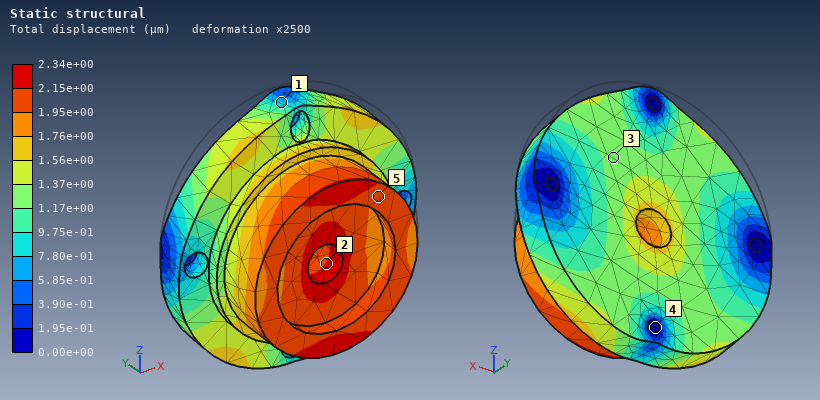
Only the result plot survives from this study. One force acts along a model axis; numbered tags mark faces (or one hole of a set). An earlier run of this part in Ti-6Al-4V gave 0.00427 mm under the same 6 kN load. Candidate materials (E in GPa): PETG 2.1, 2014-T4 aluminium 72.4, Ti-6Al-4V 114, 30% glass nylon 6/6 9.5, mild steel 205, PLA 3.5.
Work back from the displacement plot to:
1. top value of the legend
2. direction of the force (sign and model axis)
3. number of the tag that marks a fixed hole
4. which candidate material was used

2.34e+00 µm
-Z
4
mild steel
